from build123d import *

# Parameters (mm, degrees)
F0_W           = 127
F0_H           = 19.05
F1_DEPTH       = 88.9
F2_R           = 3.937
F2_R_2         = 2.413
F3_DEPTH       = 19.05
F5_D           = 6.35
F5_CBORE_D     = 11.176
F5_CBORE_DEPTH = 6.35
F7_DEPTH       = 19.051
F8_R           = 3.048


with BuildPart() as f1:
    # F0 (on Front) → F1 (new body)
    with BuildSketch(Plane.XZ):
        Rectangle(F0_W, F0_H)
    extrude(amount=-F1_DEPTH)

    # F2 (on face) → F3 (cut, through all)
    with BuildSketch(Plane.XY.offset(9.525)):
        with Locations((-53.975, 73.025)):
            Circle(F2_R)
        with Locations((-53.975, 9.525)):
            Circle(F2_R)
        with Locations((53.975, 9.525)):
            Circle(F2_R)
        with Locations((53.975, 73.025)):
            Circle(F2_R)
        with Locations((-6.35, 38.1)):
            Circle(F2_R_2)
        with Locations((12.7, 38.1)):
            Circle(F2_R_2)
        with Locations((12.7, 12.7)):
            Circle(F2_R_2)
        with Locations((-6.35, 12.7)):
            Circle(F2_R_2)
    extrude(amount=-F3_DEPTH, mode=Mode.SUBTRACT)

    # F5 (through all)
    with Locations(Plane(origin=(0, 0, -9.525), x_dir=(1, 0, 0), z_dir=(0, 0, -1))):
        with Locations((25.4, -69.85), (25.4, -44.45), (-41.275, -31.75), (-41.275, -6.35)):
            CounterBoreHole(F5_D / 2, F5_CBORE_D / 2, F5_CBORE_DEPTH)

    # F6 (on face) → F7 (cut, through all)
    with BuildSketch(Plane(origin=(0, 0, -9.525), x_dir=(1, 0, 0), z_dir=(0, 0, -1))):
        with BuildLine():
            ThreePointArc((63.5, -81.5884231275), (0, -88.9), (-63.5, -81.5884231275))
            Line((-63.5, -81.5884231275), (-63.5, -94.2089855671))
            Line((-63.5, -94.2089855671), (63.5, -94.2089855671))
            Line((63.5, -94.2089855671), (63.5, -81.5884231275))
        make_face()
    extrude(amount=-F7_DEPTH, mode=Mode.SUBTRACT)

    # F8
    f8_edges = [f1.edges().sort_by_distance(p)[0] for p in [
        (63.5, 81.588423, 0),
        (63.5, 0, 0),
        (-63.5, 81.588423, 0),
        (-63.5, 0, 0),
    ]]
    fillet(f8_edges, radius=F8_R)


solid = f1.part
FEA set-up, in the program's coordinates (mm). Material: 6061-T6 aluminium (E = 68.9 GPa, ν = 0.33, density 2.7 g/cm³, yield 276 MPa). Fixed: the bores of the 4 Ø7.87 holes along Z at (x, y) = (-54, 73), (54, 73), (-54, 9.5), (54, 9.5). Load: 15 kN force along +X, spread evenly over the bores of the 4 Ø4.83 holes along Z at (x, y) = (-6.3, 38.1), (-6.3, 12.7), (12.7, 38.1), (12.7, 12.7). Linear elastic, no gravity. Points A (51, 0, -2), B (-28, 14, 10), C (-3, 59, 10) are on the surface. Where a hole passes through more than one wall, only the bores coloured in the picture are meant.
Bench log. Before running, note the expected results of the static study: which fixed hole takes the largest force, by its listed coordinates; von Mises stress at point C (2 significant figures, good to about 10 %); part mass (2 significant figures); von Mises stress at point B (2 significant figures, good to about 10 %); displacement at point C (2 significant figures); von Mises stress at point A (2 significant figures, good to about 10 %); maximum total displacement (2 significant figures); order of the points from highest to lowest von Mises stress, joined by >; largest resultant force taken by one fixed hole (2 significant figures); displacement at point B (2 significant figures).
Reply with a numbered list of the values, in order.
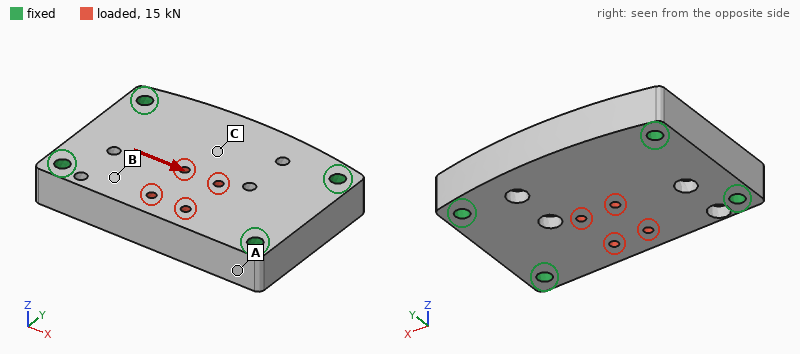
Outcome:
1. (54, 9.5)
2. 2.6 MPa
3. 540 g
4. 8.6 MPa
5. 3.0 µm
6. 5.5 MPa
7. 7.7 µm
8. B > A > C
9. 5.3 kN
10. 4.2 µm
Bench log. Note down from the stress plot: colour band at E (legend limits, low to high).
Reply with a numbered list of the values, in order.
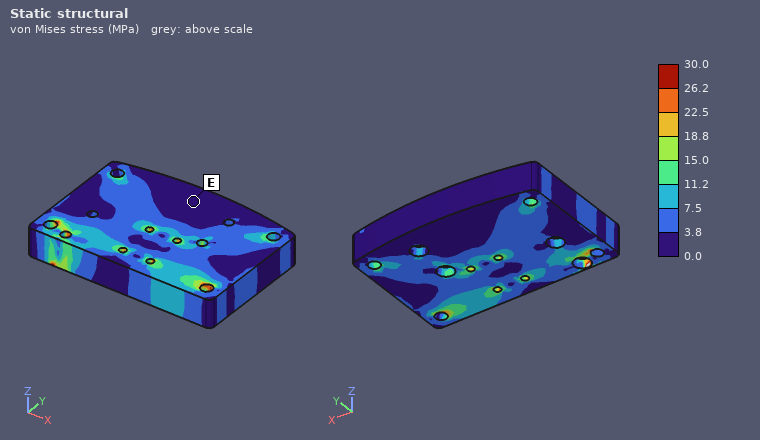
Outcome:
1. 0.0 to 3.8 MPa
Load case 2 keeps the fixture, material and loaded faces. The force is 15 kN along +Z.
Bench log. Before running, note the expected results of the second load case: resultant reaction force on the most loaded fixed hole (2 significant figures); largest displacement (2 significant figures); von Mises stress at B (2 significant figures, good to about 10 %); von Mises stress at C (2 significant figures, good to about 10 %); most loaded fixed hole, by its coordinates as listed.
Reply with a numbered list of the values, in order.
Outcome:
1. 6.2 kN
2. 76 µm
3. 14 MPa
4. 22 MPa
5. (54, 9.5)
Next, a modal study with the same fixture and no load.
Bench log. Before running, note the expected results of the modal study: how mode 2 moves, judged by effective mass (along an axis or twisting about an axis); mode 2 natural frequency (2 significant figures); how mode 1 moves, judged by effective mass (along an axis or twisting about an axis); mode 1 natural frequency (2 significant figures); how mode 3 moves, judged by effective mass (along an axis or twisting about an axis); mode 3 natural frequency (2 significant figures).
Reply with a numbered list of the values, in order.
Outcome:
1. twisting about X
2. 8200 Hz
3. along Z
4. 6000 Hz
5. along Y
6. 12 kHz
